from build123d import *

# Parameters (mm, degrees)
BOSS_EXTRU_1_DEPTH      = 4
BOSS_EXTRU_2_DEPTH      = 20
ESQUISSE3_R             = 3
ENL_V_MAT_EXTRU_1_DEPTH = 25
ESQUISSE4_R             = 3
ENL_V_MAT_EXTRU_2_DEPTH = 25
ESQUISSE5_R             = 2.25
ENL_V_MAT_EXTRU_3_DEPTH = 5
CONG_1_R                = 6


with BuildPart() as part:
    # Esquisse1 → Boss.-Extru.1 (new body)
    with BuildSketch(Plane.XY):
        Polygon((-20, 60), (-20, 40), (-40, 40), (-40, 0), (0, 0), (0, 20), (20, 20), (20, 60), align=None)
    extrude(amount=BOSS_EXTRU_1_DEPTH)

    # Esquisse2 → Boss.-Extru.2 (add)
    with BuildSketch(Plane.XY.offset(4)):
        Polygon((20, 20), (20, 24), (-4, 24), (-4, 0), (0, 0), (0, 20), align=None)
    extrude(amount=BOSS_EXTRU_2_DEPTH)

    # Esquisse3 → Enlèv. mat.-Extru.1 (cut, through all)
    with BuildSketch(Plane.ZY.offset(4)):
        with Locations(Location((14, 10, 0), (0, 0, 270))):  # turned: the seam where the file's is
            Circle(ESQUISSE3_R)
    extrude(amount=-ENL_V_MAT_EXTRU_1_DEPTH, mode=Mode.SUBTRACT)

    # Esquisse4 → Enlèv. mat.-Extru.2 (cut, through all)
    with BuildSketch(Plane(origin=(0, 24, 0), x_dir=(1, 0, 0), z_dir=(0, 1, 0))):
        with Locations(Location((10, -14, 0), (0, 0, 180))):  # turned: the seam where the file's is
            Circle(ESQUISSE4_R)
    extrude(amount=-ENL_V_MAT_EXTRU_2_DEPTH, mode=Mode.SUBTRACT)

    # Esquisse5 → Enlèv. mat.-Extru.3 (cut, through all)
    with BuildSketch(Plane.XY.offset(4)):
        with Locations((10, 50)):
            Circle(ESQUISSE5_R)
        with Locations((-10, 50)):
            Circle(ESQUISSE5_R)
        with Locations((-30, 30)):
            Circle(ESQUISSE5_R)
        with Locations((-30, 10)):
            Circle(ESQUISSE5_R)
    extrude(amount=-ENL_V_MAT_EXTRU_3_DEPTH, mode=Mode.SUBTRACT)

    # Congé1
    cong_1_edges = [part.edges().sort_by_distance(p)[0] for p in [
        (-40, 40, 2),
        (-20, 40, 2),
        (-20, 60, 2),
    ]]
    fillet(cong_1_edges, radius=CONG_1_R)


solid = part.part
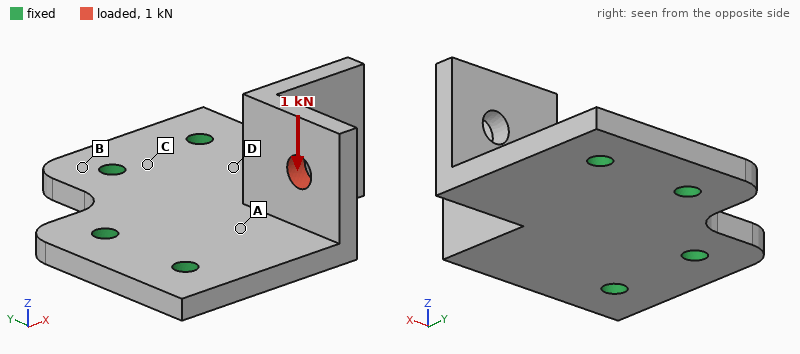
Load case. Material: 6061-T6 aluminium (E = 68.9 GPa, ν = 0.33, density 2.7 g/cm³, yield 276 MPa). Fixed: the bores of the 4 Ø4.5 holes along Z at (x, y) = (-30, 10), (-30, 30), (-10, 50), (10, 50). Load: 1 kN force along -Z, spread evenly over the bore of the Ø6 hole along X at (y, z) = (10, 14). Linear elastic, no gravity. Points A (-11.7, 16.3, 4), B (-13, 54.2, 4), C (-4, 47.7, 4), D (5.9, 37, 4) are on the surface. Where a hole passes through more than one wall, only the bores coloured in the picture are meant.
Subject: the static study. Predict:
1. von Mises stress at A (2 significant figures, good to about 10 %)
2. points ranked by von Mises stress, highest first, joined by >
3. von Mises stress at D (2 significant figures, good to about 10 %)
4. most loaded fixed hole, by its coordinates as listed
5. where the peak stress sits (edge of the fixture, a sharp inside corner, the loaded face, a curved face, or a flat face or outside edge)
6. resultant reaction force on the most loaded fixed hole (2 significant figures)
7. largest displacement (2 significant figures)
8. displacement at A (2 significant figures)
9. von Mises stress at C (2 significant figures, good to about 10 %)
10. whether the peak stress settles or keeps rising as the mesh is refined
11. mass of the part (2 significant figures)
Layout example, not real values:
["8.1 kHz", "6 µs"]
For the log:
["79 MPa", "A > D > C > B", "59 MPa", "(-30, 10)", "edge of the fixture", "780 N", "0.46 mm", "0.11 mm", "40 MPa", "keeps rising", "38 g"]
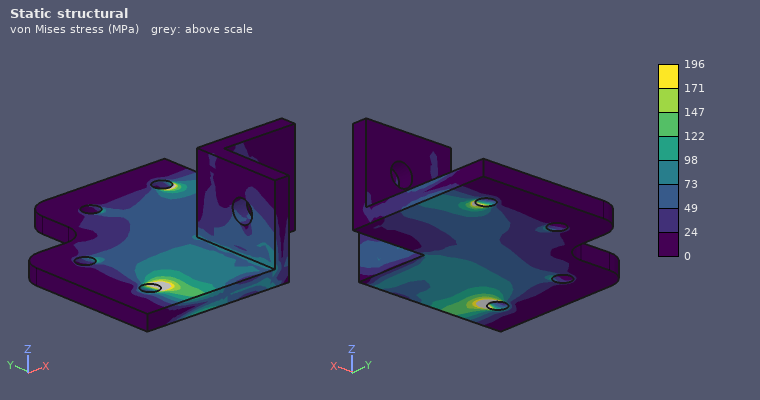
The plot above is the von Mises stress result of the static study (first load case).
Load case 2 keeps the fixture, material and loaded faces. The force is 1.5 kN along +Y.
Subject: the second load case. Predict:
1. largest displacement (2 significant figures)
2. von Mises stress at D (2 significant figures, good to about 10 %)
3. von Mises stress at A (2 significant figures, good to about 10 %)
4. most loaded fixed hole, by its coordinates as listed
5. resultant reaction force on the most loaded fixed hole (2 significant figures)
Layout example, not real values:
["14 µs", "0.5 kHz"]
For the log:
["0.41 mm", "48 MPa", "95 MPa", "(-10, 50)", "740 N"]
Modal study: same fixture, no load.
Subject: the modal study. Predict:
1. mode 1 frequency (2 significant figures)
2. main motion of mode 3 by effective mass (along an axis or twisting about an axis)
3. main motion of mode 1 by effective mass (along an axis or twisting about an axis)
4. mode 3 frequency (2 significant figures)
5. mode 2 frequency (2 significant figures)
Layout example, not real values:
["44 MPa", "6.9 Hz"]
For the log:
["2500 Hz", "along Z", "along Z", "6600 Hz", "4900 Hz"]
